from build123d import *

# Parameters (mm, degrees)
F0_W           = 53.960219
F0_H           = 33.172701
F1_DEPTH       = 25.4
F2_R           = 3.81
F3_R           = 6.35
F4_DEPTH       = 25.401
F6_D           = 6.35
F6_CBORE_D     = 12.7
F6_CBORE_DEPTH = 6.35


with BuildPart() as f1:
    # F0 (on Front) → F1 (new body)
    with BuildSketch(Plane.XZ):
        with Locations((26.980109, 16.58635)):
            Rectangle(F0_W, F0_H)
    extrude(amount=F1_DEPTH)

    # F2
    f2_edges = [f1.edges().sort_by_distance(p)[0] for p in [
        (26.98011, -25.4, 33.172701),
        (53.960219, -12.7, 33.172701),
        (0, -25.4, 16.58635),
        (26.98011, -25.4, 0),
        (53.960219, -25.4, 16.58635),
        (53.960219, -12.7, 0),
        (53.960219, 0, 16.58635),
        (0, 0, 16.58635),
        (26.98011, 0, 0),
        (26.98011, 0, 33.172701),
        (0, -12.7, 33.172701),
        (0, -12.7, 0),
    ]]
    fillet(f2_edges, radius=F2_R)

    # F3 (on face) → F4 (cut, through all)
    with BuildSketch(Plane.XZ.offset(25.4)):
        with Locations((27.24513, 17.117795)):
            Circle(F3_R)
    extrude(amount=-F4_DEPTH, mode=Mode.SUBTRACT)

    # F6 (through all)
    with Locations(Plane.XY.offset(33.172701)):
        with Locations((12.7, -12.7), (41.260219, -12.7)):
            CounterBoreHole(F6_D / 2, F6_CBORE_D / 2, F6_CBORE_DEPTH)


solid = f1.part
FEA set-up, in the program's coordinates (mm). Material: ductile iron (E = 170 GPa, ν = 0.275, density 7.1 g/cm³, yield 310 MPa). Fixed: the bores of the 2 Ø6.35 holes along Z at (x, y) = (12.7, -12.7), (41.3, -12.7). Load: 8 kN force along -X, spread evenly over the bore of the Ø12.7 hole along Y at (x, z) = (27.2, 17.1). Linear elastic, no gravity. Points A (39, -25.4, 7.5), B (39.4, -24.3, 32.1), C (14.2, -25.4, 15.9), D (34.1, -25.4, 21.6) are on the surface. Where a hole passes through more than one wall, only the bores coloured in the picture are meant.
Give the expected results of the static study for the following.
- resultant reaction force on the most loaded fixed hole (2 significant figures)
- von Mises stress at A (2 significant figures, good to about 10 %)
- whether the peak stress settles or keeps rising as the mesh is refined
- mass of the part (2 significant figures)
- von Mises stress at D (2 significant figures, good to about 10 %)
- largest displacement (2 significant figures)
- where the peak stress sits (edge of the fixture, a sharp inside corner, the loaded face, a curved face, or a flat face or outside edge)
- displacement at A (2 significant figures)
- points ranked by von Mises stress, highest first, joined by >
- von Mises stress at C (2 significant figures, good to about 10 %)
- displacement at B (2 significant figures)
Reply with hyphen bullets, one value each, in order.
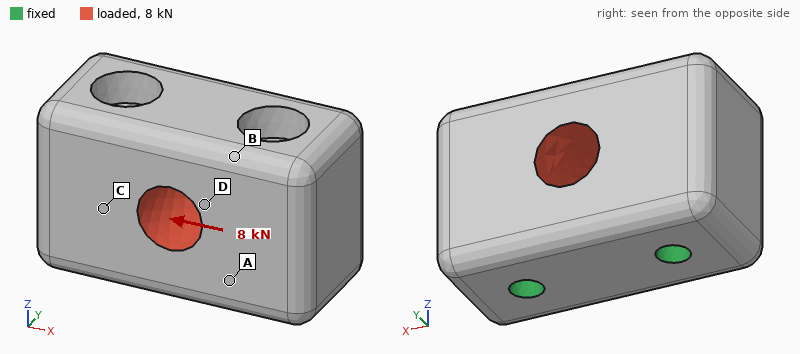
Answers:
- 4.0 kN
- 3.6 MPa
- keeps rising
- 270 g
- 8.9 MPa
- 0.85 µm
- edge of the fixture
- 0.33 µm
- D > C > A > B
- 5.7 MPa
- 0.49 µm
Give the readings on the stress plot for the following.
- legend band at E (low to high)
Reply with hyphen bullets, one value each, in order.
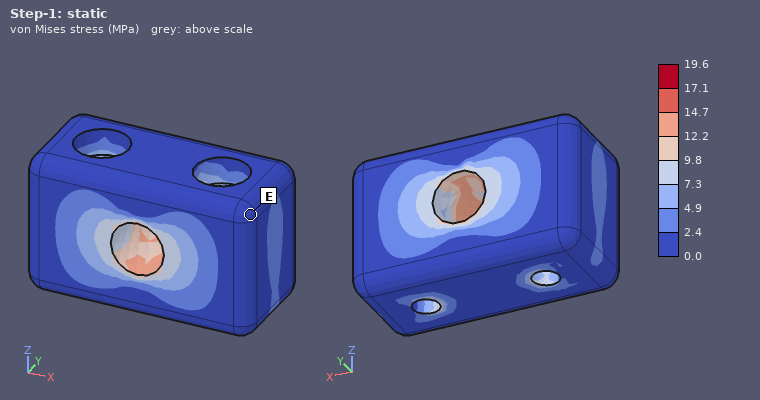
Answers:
- 0.0 to 2.4 MPa
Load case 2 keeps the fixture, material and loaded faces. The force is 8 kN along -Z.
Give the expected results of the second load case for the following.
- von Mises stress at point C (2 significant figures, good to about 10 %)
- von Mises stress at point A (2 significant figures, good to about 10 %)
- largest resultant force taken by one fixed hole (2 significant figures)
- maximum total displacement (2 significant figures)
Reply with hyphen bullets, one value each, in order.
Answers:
- 5.8 MPa
- 5.2 MPa
- 4.1 kN
- 1.6 µm
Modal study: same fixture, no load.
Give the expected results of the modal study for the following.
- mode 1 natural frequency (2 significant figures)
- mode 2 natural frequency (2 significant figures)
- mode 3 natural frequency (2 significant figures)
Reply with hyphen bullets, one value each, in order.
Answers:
- 31 kHz
- 32 kHz
- 33 kHz
